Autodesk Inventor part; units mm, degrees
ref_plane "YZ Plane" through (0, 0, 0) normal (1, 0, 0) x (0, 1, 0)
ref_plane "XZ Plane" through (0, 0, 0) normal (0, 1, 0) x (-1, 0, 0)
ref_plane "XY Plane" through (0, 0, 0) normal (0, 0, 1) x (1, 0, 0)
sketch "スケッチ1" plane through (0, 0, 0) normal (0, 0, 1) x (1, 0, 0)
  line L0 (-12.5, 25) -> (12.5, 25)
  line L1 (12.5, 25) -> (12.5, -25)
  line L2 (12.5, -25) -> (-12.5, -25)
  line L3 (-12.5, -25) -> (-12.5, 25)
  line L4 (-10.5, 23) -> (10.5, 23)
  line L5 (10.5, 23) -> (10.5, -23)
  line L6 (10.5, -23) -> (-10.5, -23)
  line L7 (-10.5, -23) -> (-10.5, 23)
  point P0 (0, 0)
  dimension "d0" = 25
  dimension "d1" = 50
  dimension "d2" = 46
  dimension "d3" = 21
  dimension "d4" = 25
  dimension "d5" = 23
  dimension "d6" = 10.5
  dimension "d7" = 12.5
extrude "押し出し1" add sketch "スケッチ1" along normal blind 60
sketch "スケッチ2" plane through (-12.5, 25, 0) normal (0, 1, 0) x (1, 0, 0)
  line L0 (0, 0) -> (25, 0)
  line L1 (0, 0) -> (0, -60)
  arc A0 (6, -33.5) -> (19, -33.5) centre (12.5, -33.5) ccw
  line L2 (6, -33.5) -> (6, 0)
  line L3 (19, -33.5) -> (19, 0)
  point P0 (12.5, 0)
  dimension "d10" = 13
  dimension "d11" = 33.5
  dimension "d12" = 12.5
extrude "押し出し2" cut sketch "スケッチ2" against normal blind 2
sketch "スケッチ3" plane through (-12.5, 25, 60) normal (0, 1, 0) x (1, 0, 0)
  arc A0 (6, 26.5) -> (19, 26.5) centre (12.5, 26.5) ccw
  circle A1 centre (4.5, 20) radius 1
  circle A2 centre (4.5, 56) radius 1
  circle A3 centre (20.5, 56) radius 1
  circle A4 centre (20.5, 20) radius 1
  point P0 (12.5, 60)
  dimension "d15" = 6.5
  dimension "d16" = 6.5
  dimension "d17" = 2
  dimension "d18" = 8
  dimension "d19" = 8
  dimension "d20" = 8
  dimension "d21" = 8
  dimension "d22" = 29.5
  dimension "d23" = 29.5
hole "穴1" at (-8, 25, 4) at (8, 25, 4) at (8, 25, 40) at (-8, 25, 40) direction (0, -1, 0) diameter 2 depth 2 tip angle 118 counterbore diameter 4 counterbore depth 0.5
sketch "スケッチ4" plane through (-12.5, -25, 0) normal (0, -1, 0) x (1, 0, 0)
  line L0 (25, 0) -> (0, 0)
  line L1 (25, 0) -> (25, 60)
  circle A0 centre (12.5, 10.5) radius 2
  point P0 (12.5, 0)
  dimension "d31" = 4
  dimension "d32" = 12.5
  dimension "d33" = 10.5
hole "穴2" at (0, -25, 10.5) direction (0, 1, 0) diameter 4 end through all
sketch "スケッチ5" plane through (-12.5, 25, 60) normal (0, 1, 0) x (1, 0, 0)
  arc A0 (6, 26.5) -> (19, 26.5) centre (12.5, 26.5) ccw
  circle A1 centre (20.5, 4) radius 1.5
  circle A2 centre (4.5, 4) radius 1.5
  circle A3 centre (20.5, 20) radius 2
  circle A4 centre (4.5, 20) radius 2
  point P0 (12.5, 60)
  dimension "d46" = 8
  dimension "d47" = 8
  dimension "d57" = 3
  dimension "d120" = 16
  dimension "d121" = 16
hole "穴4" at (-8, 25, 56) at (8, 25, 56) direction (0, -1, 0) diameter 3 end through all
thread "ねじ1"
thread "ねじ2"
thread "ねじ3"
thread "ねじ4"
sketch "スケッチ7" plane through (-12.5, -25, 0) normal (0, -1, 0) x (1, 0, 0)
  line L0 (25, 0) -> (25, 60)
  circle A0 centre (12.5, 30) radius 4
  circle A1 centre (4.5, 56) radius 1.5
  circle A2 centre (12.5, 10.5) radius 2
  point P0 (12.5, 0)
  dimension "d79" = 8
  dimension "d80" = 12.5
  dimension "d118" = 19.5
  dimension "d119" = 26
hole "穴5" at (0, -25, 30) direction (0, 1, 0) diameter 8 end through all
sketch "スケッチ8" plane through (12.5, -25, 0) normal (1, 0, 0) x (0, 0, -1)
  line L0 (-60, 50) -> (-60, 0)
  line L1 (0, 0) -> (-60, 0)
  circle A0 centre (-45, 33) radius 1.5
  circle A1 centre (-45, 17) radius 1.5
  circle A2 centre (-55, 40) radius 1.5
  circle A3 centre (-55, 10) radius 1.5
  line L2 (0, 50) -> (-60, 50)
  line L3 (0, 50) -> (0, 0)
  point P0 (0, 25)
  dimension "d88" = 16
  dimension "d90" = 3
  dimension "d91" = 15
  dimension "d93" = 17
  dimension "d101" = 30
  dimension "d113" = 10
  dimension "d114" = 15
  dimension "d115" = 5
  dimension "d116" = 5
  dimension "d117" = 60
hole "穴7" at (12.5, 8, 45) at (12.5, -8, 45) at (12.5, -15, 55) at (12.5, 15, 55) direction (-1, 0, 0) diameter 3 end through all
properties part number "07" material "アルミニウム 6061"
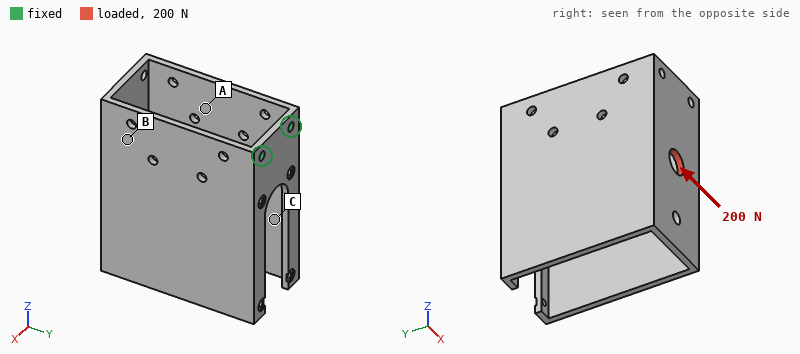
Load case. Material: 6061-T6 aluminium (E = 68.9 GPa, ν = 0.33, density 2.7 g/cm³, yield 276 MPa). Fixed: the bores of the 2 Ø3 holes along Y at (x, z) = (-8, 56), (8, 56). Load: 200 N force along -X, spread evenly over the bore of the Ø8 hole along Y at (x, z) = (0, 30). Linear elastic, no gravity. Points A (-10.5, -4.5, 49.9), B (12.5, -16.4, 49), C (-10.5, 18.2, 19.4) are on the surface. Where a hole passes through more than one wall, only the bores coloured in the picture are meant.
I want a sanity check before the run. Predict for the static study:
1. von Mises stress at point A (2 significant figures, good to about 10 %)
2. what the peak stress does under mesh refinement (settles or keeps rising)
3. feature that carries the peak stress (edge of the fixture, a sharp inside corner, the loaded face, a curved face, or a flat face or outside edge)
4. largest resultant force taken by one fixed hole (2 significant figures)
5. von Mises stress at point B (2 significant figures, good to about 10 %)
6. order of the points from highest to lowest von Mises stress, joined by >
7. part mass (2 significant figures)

30 MPa
keeps rising
edge of the fixture
470 N
59 MPa
B > A > C
42 g
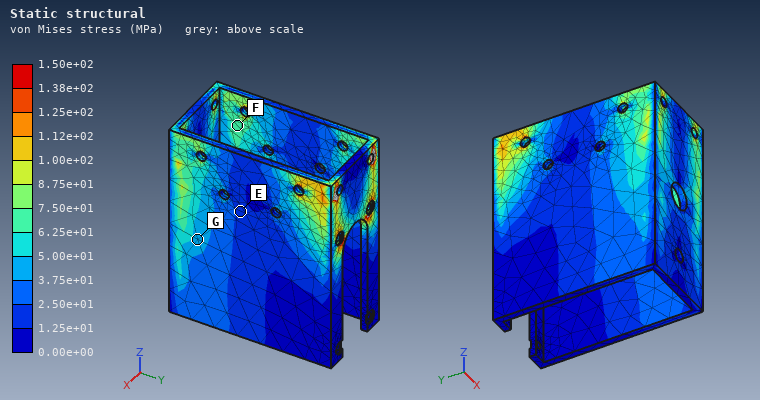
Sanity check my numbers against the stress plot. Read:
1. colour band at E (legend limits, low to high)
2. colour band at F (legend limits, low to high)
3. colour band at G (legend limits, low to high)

1.25e+01 to 2.50e+01 MPa
6.25e+01 to 7.50e+01 MPa
3.75e+01 to 5.00e+01 MPa
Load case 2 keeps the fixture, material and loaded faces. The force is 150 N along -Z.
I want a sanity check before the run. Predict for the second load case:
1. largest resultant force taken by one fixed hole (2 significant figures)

75 N
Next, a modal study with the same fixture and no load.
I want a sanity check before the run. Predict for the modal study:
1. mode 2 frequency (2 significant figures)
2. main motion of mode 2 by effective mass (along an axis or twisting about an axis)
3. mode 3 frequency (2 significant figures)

570 Hz
along X
1100 Hz
